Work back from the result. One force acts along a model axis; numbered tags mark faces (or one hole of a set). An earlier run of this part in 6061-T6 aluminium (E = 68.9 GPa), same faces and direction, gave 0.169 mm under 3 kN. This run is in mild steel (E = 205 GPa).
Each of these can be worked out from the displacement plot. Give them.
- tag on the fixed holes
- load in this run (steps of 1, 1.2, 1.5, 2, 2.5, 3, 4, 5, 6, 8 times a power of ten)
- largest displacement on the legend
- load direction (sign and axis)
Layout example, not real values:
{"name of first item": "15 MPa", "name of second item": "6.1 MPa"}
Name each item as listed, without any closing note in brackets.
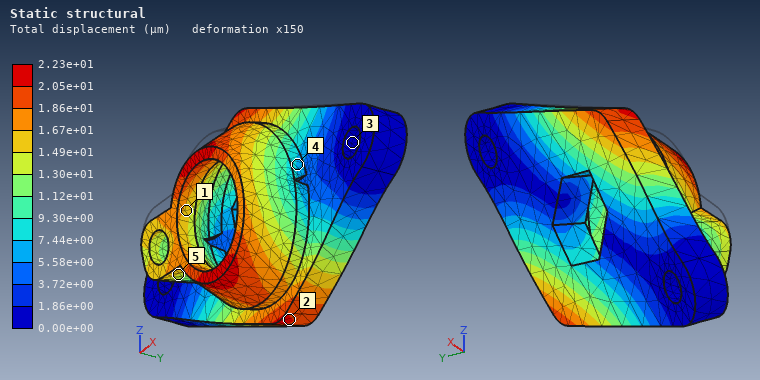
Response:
{"tag on the fixed holes": "3", "load in this run": "1.2 kN", "largest displacement on the legend": "2.23e+01 µm", "load direction": "-Z"}
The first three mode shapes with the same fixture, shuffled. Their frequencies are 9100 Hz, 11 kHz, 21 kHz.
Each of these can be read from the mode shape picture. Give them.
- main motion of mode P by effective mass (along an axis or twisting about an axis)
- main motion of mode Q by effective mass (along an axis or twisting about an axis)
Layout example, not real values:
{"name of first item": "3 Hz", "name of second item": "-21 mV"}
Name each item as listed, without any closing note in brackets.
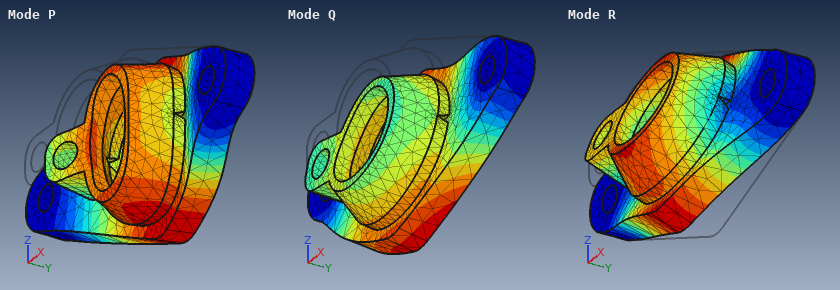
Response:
{"main motion of mode P by effective mass": "along Y", "main motion of mode Q by effective mass": "along Z"}
